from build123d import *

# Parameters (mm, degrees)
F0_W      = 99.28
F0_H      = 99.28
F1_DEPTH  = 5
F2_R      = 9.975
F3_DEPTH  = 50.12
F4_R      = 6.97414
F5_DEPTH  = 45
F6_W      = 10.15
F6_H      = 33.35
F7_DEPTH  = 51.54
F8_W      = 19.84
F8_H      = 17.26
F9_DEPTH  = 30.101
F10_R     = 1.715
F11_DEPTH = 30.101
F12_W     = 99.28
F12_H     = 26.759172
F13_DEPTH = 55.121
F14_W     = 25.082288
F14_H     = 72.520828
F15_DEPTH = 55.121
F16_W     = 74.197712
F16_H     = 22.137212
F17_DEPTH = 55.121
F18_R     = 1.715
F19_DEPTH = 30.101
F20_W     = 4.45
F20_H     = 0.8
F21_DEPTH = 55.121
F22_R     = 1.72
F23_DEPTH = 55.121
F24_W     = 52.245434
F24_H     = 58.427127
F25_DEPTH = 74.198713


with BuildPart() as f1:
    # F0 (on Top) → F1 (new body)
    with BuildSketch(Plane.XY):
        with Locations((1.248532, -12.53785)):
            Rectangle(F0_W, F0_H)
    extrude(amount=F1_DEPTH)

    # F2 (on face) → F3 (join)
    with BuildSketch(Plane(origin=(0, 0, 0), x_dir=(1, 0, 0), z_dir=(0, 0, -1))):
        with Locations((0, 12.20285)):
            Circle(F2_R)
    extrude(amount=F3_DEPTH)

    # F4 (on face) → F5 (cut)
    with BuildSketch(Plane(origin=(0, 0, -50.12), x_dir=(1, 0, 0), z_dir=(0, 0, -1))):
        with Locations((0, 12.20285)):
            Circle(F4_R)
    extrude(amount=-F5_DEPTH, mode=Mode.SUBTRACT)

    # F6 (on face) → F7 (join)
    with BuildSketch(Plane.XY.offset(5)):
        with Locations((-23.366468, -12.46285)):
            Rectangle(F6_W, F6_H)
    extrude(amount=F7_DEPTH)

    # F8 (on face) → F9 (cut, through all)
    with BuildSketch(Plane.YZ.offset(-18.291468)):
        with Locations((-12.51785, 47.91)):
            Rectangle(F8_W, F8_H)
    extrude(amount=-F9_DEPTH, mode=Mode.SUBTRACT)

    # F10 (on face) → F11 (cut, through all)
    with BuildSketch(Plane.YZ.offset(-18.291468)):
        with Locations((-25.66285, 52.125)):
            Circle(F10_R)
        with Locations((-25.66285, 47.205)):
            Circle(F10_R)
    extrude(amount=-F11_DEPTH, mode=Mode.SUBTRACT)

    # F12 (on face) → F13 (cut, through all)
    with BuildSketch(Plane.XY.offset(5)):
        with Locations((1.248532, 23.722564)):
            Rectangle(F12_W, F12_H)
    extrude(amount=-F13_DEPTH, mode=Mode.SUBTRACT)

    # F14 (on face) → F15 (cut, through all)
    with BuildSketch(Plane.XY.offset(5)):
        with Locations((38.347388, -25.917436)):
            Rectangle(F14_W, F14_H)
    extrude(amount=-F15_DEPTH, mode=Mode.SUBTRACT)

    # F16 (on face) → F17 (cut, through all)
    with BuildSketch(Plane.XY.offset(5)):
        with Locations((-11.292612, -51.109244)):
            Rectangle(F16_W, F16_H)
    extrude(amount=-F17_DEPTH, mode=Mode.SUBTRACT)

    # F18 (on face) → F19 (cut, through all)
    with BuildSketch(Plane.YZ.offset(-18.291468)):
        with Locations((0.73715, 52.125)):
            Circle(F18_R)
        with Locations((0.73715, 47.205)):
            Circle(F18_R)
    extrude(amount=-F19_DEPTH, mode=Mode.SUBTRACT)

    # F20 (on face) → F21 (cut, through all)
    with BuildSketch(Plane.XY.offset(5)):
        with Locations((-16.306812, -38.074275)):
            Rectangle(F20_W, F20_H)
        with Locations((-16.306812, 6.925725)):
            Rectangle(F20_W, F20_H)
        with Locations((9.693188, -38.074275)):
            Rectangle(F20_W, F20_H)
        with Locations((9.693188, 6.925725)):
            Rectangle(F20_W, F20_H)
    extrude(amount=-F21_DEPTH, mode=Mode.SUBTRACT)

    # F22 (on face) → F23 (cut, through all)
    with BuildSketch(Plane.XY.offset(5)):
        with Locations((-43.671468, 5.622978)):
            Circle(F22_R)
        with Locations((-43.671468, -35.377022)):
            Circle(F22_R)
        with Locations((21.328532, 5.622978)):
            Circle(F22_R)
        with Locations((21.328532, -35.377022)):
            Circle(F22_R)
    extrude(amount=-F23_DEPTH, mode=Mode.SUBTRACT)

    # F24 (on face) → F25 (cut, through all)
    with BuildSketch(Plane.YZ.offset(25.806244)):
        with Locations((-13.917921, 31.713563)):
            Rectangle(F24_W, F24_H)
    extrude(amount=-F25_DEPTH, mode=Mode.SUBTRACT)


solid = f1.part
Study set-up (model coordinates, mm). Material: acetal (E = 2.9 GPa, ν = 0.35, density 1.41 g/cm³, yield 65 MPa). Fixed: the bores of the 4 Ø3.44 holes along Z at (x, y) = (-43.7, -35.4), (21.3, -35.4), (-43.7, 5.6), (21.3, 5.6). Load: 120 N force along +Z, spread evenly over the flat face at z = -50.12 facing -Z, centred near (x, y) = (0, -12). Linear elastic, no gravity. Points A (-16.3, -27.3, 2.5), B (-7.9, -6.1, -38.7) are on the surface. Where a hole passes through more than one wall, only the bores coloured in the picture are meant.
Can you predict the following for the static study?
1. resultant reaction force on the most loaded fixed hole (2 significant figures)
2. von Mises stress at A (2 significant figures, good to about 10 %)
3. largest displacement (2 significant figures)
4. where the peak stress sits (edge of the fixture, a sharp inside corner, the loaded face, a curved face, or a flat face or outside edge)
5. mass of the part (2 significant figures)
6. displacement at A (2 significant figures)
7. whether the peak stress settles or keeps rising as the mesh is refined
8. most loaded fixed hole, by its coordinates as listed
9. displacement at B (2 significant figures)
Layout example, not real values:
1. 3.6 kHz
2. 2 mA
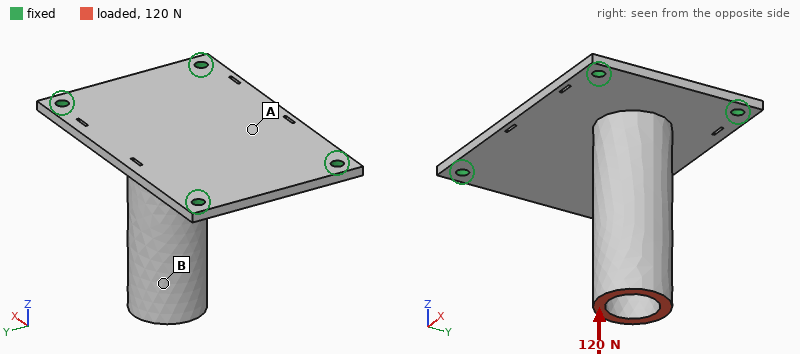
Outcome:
1. 50 N
2. 7.0 MPa
3. 1.2 mm
4. edge of the fixture
5. 25 g
6. 0.62 mm
7. keeps rising
8. (21.3, 5.6)
9. 1.00 mm
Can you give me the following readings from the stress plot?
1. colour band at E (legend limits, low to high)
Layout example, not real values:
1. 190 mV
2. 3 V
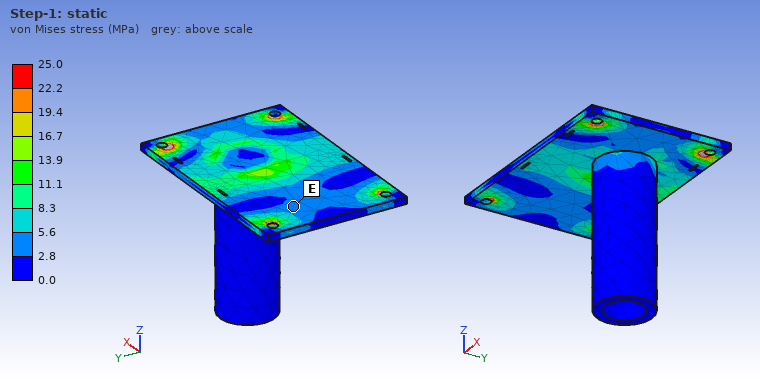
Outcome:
1. 2.8 to 5.6 MPa
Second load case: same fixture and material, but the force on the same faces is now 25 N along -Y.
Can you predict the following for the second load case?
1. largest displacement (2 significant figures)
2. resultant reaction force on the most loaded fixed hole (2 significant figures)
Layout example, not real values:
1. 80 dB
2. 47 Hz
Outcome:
1. 1.1 mm
2. 31 N
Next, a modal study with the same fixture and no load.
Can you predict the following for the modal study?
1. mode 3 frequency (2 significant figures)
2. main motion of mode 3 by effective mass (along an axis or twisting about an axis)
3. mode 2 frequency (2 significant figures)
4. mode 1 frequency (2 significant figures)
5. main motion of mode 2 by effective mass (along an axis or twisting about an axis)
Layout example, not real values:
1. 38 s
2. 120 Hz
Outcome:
1. 650 Hz
2. along Z
3. 370 Hz
4. 340 Hz
5. along Y
